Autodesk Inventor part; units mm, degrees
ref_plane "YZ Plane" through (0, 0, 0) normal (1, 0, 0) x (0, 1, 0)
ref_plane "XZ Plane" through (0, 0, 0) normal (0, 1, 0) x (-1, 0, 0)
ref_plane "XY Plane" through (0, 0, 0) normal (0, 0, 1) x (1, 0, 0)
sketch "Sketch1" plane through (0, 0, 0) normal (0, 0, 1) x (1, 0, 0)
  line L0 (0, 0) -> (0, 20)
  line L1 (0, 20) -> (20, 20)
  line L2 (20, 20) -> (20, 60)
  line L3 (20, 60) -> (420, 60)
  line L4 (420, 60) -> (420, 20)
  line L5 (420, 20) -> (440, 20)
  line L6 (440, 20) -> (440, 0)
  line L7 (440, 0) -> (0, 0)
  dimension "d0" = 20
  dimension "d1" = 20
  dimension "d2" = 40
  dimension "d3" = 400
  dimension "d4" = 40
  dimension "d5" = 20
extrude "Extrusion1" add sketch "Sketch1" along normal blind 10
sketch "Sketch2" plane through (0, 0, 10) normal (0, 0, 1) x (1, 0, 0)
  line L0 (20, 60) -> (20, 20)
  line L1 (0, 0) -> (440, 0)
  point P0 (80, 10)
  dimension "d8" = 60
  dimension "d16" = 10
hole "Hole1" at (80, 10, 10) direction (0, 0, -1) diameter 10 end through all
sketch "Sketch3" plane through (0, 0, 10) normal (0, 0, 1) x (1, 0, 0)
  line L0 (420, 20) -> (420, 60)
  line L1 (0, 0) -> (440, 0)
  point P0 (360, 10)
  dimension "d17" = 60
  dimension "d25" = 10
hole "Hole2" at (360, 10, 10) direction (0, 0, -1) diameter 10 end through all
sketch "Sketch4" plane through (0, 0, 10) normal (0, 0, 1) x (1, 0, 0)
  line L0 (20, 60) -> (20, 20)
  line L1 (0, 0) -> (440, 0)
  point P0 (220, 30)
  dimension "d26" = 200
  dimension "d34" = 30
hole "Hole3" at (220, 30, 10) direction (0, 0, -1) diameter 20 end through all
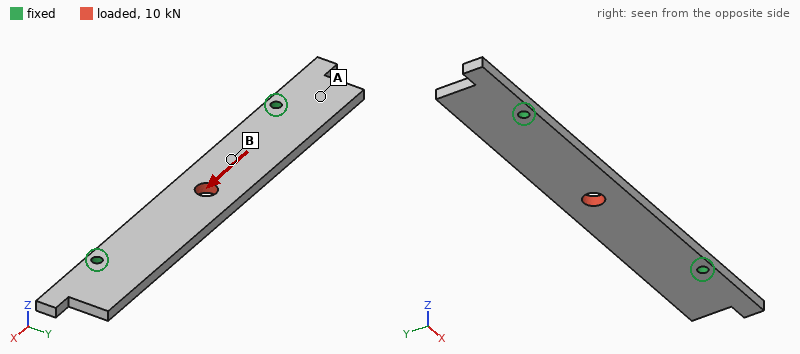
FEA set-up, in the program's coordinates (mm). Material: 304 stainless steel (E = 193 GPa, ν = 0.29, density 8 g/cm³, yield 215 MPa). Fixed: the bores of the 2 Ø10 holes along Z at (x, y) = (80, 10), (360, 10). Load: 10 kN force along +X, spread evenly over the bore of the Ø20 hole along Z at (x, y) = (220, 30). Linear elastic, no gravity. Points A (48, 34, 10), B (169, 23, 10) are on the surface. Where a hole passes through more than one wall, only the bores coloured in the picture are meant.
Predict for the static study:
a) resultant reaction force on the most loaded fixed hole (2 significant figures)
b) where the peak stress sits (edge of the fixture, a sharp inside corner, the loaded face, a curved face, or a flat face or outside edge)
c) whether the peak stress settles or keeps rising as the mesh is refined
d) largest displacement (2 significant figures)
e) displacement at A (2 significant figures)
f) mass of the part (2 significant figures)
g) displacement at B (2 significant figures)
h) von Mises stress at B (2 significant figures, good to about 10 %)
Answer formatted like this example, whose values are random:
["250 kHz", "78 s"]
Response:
["5.0 kN", "edge of the fixture", "keeps rising", "9.4 µm", "4.7 µm", "1.9 kg", "6.9 µm", "10 MPa"]
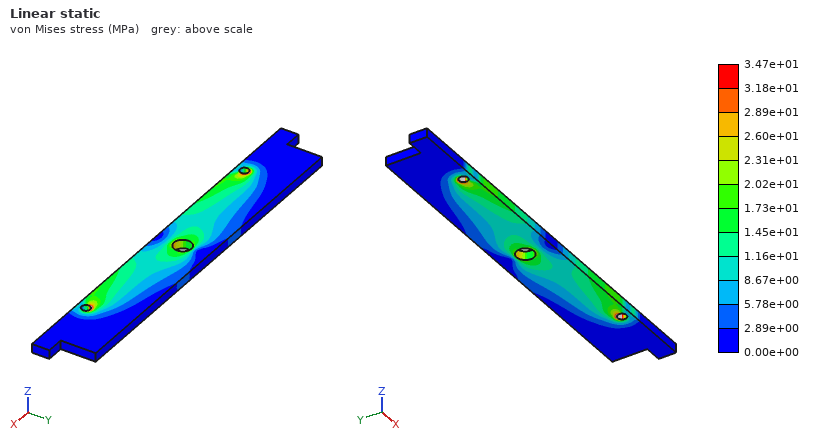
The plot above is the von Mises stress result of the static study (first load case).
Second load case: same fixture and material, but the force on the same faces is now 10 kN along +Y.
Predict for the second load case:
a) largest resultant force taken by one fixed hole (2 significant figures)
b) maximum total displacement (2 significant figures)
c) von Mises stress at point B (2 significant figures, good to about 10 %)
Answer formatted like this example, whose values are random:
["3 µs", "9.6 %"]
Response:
["8.6 kN", "82 µm", "20 MPa"]
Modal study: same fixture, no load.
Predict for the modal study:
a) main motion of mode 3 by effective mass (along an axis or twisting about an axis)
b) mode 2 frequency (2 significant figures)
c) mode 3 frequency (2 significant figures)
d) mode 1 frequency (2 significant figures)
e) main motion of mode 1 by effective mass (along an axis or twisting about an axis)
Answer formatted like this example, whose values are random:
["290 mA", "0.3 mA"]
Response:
["along Z", "1400 Hz", "1500 Hz", "580 Hz", "along Z"]
